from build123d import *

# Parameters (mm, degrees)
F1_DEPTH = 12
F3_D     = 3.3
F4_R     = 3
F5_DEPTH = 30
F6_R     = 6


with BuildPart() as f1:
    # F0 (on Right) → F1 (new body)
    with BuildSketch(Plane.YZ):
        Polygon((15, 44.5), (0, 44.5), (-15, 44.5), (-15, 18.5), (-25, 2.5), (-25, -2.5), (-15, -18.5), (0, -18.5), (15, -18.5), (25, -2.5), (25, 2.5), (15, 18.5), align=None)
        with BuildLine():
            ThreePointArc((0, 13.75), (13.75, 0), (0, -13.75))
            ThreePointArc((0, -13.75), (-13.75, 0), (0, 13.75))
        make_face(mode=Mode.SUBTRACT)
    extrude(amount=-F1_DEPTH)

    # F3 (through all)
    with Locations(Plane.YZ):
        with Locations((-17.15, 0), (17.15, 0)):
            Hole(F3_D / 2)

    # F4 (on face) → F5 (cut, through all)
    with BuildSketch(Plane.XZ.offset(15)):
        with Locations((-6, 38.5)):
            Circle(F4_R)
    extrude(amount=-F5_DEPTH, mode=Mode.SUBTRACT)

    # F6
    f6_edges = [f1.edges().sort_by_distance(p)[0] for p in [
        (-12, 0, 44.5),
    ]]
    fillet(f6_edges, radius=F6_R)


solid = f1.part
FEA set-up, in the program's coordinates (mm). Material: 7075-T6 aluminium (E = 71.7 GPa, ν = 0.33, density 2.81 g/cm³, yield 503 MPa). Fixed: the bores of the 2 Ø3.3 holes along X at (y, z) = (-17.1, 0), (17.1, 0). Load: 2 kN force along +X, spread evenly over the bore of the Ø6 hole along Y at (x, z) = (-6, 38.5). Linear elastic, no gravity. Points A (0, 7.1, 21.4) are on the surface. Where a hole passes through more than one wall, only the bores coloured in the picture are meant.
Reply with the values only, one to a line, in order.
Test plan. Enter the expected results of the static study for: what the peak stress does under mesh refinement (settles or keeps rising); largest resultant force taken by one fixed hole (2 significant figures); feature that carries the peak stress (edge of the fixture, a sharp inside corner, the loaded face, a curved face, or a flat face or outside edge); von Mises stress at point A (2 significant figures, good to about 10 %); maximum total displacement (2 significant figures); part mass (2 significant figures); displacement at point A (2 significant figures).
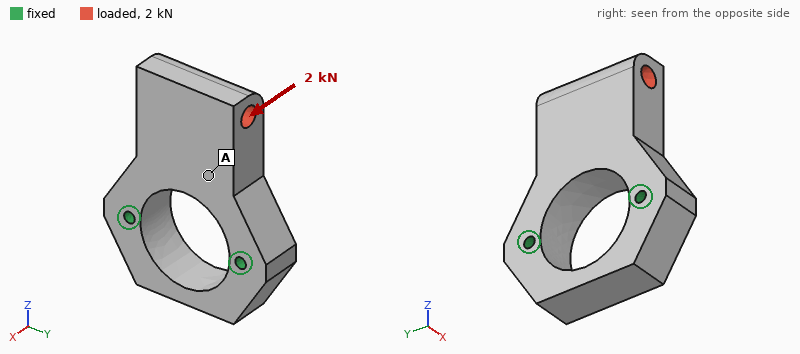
keeps rising
1.0 kN
edge of the fixture
44 MPa
0.29 mm
54 g
0.11 mm
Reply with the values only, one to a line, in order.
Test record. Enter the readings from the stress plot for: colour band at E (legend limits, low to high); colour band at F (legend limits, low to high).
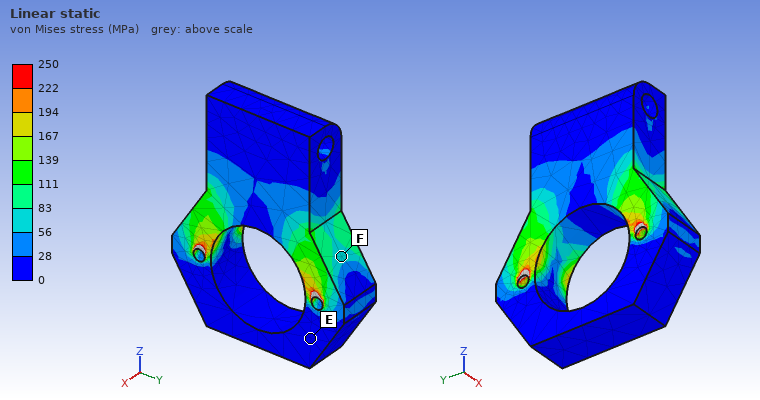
0 to 28 MPa
56 to 83 MPa
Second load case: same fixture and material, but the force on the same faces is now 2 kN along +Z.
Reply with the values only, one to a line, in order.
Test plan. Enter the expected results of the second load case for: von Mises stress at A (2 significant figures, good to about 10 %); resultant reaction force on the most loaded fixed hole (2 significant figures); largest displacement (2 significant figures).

5.9 MPa
1.1 kN
5.9 µm
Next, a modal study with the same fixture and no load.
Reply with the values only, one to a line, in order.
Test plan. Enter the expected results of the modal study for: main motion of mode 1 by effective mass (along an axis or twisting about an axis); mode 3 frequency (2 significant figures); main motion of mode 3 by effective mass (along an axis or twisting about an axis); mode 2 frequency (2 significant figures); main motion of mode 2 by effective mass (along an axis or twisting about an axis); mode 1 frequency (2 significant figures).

along X
13 kHz
twisting about Z
11 kHz
along Y
3900 Hz
